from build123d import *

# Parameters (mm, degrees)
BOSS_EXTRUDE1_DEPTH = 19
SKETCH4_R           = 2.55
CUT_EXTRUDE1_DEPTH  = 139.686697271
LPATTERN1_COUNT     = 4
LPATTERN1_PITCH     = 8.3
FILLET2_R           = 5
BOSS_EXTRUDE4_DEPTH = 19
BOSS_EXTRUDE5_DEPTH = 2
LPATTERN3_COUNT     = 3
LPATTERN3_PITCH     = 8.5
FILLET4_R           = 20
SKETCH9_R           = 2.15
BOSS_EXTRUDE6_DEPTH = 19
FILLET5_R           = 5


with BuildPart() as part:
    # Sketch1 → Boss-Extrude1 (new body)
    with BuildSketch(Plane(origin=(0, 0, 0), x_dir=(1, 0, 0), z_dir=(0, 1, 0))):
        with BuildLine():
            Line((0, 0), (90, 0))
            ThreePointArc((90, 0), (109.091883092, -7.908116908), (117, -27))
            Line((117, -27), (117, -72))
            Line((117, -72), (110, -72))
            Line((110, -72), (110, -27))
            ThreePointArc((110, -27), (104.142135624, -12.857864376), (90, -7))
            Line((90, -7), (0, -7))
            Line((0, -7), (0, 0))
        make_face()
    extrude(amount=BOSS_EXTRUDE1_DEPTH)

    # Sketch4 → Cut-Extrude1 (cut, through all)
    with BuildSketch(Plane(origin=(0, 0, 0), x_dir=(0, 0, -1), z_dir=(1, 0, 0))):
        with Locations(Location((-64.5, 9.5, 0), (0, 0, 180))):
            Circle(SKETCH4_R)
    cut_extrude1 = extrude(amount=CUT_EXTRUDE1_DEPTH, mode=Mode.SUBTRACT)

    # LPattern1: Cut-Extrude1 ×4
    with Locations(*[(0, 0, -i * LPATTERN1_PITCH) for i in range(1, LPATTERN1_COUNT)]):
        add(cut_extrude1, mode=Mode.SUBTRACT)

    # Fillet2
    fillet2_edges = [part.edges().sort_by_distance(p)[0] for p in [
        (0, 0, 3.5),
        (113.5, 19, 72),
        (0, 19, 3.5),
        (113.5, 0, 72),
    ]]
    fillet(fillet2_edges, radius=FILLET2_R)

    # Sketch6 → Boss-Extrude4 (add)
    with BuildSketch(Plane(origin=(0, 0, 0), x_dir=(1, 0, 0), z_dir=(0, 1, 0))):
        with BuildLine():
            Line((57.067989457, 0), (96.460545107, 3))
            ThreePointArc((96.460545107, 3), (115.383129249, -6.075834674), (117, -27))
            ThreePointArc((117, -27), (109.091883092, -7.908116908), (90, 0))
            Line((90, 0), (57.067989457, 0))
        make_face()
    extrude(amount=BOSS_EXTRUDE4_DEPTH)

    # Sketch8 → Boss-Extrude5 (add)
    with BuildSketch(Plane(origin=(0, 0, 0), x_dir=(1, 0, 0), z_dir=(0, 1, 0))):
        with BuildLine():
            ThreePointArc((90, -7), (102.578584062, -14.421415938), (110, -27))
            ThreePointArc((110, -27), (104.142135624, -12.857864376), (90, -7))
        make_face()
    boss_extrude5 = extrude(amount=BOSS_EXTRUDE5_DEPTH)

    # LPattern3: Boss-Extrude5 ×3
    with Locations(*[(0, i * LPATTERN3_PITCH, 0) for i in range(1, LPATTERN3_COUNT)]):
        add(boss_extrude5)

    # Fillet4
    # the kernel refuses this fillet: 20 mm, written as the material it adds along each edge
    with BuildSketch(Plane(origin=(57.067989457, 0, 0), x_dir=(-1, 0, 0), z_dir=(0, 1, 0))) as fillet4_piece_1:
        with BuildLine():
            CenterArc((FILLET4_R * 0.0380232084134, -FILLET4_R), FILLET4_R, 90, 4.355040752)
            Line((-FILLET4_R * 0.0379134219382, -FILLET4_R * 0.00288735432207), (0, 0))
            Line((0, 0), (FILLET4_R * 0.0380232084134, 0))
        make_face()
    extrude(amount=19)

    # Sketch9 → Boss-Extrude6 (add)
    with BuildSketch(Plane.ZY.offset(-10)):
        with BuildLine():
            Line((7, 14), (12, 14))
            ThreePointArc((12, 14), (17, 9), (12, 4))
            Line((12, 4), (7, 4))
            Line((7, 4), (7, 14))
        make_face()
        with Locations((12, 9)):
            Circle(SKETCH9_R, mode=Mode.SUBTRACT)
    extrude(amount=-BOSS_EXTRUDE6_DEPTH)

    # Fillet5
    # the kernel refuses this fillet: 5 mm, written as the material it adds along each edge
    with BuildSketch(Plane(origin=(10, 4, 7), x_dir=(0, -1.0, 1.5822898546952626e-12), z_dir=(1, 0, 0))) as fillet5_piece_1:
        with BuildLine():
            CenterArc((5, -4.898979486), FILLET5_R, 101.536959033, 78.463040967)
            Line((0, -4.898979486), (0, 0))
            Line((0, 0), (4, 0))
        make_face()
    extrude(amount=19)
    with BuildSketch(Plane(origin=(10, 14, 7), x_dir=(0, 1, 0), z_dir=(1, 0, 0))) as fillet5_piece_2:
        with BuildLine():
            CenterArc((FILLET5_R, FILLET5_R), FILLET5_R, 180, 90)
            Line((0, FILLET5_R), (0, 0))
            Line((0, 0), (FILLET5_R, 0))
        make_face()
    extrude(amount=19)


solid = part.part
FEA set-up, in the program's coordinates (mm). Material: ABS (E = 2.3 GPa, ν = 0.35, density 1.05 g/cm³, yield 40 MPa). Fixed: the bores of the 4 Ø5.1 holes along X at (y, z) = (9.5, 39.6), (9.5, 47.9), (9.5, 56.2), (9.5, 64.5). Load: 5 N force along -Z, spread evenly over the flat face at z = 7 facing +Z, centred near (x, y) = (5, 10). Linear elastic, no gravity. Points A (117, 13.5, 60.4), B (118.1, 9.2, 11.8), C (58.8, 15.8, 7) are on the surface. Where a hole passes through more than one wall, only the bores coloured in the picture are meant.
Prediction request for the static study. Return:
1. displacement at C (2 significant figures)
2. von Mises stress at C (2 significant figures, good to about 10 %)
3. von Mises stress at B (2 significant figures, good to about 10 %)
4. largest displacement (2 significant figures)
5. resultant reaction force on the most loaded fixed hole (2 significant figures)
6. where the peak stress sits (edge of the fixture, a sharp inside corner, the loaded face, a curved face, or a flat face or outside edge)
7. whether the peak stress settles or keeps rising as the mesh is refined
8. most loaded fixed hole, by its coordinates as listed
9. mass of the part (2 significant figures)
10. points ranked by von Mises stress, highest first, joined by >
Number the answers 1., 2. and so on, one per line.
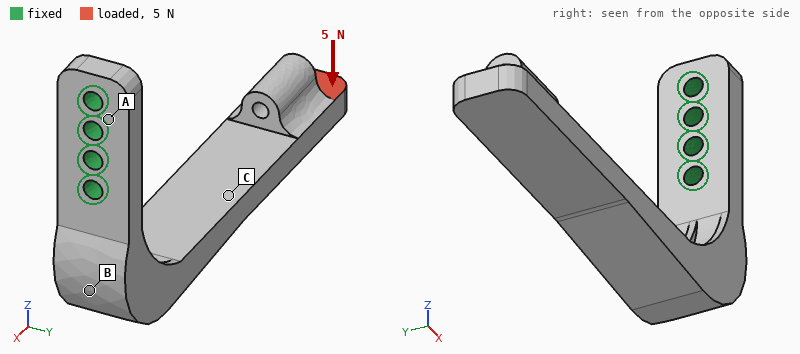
1. 0.58 mm
2. 1.6 MPa
3. 0.79 MPa
4. 1.7 mm
5. 16 N
6. edge of the fixture
7. keeps rising
8. (9.5, 39.6)
9. 30 g
10. C > B > A
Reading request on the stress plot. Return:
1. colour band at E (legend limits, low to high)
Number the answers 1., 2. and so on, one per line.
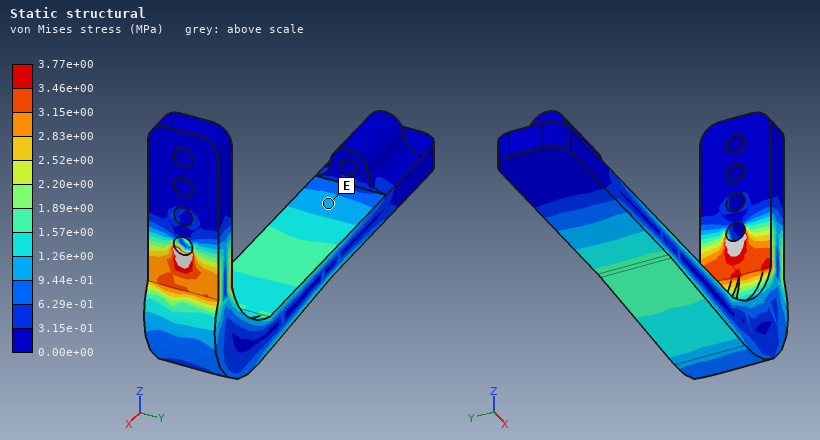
1. 9.44e-01 to 1.26e+00 MPa
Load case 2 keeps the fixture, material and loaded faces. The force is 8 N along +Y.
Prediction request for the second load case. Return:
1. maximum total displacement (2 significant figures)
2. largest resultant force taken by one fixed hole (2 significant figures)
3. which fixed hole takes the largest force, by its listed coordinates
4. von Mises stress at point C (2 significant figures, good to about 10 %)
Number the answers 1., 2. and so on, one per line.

1. 1.5 mm
2. 19 N
3. (9.5, 39.6)
4. 0.65 MPa
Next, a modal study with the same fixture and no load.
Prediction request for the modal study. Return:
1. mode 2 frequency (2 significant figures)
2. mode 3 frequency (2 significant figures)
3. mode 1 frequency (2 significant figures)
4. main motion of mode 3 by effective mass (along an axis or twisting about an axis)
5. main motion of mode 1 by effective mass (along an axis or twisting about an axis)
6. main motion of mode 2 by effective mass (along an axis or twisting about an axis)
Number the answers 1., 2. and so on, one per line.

1. 150 Hz
2. 450 Hz
3. 110 Hz
4. along X
5. along Z
6. along Y
